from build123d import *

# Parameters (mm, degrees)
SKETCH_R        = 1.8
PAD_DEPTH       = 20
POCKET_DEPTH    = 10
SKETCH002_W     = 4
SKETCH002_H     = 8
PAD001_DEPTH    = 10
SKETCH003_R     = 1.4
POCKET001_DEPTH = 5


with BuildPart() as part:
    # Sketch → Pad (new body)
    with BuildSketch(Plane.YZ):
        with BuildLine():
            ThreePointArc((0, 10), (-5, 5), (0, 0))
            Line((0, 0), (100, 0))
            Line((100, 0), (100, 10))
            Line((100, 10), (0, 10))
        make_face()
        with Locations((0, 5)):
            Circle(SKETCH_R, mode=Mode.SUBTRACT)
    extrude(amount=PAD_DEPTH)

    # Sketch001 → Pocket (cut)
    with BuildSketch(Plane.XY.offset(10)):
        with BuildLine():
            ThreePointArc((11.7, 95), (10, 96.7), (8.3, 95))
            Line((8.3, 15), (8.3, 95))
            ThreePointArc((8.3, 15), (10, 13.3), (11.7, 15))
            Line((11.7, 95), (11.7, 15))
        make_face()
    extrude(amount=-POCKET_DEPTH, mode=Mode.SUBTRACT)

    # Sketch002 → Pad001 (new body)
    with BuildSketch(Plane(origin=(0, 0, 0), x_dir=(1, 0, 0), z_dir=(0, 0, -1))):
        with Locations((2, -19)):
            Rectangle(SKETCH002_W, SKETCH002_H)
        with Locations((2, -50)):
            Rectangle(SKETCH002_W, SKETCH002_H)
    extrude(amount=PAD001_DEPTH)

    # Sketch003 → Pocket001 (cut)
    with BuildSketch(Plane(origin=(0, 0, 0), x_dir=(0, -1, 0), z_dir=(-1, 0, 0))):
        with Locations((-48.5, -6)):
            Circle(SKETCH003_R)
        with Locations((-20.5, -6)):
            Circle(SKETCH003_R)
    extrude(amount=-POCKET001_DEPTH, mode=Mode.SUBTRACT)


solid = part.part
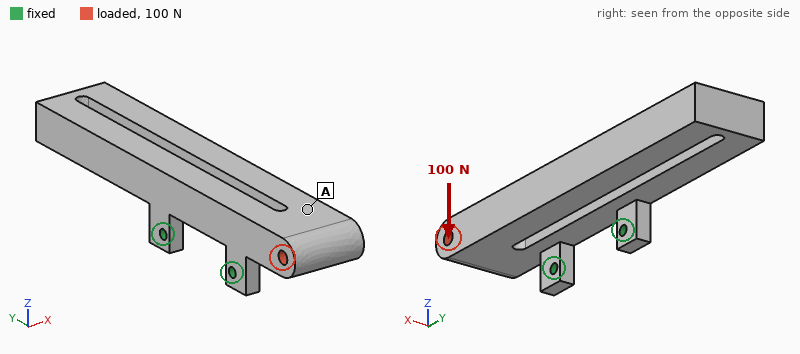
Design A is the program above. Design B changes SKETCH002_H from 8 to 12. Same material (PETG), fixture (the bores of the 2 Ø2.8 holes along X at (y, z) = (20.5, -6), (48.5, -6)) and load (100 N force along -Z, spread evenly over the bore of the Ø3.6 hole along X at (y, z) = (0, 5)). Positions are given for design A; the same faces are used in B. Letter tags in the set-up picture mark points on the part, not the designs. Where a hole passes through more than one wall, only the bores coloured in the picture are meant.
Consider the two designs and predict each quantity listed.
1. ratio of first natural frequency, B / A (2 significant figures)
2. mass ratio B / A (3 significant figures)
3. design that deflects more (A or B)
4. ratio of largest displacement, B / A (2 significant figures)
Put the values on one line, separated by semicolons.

1.1; 1.02; A; 0.81
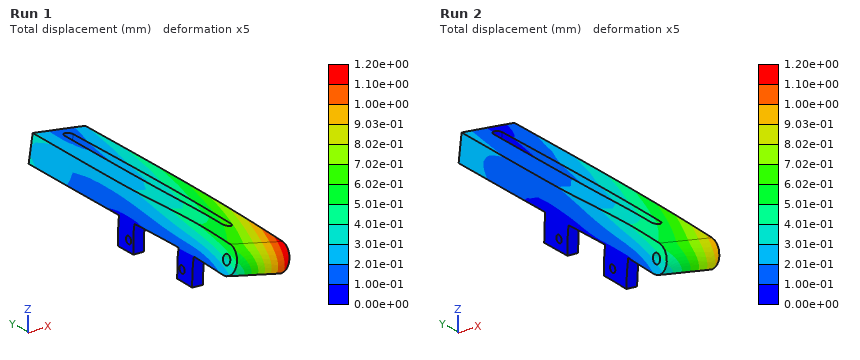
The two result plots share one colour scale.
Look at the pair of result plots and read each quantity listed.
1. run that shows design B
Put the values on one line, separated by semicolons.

Run 2
